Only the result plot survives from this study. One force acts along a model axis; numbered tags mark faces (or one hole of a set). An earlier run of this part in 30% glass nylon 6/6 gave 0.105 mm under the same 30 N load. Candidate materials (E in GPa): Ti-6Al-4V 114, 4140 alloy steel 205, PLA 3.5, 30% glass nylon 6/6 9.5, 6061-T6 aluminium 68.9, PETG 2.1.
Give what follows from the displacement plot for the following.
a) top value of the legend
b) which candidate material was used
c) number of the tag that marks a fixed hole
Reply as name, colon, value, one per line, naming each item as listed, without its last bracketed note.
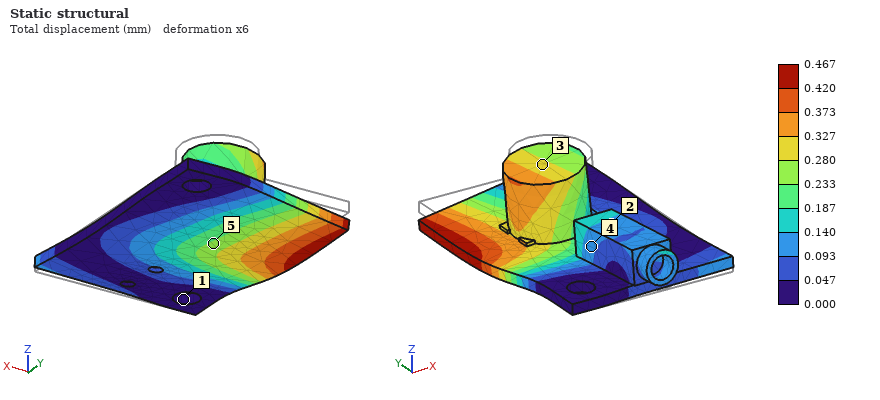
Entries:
top value of the legend: 0.467 mm
which candidate material was used: PETG
number of the tag that marks a fixed hole: 1
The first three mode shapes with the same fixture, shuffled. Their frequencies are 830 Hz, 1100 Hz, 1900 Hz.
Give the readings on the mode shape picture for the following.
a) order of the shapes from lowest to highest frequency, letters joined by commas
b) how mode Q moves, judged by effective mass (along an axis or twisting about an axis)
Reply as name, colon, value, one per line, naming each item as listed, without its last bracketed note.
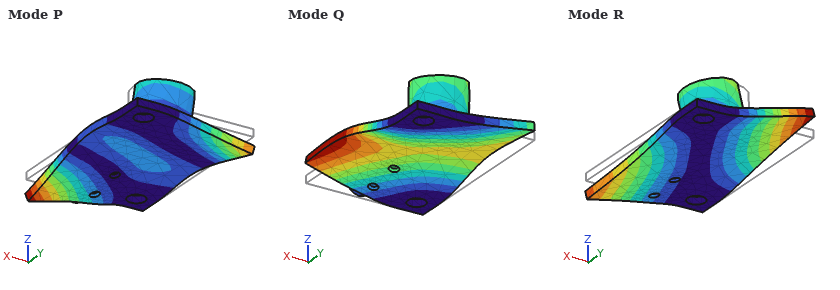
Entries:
order of the shapes from lowest to highest frequency, letters joined by commas: R, Q, P
how mode Q moves, judged by effective mass: along Z
